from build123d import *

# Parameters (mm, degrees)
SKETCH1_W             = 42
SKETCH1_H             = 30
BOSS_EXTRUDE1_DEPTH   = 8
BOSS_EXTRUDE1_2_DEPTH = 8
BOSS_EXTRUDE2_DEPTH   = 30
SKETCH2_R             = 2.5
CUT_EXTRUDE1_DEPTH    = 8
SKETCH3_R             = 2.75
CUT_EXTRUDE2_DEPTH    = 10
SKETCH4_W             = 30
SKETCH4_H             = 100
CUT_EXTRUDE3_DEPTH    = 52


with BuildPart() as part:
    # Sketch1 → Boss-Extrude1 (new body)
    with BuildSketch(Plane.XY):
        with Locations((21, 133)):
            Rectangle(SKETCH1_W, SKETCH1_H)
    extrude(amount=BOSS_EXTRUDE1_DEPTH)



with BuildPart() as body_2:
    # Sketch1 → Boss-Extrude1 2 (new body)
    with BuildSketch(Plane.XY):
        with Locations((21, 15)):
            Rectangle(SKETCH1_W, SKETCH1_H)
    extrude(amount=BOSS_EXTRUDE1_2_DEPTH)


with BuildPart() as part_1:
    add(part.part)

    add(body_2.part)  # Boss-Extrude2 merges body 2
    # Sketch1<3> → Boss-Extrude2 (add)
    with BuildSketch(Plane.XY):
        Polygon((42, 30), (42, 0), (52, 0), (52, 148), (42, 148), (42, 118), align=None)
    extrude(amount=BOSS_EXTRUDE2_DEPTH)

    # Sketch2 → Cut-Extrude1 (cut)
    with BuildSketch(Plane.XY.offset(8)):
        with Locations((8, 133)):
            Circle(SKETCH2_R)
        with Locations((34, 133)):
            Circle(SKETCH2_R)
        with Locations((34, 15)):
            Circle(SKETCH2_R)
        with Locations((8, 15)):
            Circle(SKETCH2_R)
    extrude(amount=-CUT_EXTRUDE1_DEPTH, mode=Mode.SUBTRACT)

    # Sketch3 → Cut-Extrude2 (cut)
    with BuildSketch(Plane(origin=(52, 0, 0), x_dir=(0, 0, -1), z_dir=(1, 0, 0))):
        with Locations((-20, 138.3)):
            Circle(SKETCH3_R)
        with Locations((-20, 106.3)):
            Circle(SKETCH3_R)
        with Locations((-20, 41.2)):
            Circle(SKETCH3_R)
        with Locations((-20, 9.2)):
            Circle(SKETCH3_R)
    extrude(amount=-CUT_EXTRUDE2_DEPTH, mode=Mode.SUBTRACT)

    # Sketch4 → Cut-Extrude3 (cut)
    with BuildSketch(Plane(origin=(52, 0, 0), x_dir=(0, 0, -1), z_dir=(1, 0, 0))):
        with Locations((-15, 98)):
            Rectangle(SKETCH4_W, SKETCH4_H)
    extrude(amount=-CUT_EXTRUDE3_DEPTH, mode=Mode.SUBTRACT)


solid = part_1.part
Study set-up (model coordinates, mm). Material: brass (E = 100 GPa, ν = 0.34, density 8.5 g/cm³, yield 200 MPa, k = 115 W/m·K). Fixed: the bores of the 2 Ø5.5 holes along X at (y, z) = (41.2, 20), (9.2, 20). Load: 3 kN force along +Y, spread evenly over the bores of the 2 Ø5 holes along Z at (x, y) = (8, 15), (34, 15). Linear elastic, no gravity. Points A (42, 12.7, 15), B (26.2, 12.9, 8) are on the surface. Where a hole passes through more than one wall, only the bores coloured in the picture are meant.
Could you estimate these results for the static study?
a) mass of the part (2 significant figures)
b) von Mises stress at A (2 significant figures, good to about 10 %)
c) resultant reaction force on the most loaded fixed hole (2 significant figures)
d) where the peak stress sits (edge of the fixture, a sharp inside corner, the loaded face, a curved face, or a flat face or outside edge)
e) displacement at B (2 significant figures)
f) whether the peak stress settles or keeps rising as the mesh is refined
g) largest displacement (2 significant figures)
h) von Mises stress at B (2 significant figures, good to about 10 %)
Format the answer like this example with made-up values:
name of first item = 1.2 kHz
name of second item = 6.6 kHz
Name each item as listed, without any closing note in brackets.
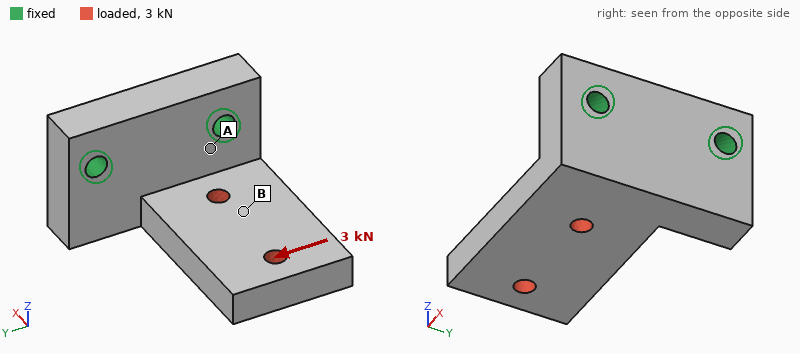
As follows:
mass of the part = 200 g
von Mises stress at A = 69 MPa
resultant reaction force on the most loaded fixed hole = 3.0 kN
where the peak stress sits = edge of the fixture
displacement at B = 0.046 mm
whether the peak stress settles or keeps rising as the mesh is refined = keeps rising
largest displacement = 0.11 mm
von Mises stress at B = 26 MPa
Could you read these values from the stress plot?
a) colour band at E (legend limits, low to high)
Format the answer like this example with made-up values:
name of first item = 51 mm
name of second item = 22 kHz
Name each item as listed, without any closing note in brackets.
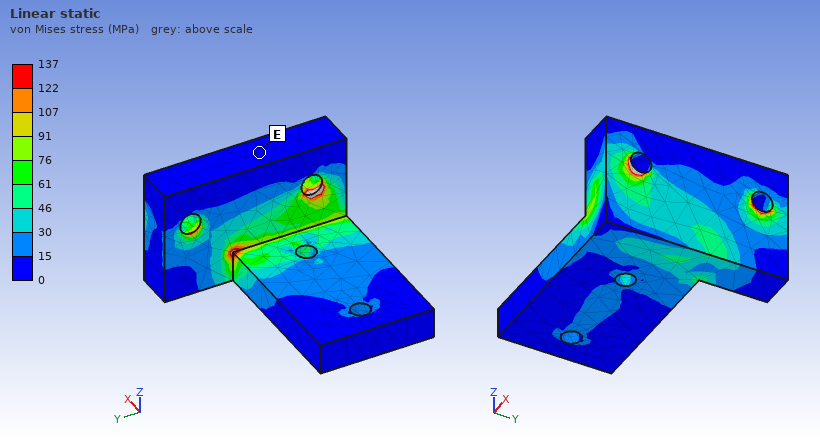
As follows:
colour band at E = 0 to 15 MPa
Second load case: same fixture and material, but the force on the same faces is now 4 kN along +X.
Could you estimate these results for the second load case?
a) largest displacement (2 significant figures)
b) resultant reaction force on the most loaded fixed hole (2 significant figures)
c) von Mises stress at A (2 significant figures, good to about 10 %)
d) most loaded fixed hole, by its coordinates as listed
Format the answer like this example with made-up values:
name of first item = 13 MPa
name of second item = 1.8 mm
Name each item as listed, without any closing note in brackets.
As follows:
largest displacement = 99 µm
resultant reaction force on the most loaded fixed hole = 3.1 kN
von Mises stress at A = 80 MPa
most loaded fixed hole, by its coordinates as listed = (9.2, 20)
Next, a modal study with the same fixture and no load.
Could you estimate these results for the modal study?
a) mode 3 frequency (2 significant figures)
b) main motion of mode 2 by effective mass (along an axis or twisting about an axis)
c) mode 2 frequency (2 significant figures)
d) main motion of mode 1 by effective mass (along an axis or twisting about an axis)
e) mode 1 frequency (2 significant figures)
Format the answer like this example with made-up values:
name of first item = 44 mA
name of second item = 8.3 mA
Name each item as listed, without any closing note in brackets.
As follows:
mode 3 frequency = 5900 Hz
main motion of mode 2 by effective mass = along Y
mode 2 frequency = 3500 Hz
main motion of mode 1 by effective mass = along Z
mode 1 frequency = 1700 Hz
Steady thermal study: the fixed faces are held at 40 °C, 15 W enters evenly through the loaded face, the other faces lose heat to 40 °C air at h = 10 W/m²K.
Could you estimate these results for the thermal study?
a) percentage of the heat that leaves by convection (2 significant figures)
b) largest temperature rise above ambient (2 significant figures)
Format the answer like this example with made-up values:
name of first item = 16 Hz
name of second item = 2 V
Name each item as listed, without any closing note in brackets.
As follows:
percentage of the heat that leaves by convection = 3.8 %
largest temperature rise above ambient = 20 K
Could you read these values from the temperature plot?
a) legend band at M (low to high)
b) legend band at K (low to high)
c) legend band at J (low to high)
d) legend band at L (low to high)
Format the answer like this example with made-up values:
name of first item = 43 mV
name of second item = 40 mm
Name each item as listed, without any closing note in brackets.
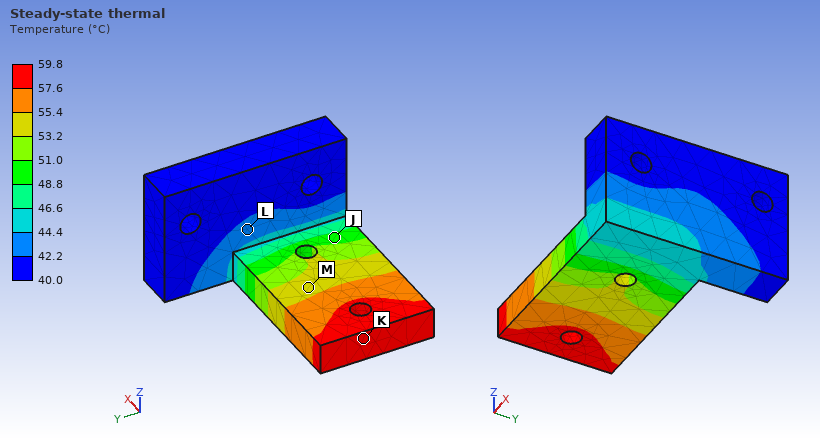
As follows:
legend band at M = 53.2 to 55.4 °C
legend band at K = 57.6 to 59.8 °C
legend band at J = 48.8 to 51.0 °C
legend band at L = 42.2 to 44.4 °C
